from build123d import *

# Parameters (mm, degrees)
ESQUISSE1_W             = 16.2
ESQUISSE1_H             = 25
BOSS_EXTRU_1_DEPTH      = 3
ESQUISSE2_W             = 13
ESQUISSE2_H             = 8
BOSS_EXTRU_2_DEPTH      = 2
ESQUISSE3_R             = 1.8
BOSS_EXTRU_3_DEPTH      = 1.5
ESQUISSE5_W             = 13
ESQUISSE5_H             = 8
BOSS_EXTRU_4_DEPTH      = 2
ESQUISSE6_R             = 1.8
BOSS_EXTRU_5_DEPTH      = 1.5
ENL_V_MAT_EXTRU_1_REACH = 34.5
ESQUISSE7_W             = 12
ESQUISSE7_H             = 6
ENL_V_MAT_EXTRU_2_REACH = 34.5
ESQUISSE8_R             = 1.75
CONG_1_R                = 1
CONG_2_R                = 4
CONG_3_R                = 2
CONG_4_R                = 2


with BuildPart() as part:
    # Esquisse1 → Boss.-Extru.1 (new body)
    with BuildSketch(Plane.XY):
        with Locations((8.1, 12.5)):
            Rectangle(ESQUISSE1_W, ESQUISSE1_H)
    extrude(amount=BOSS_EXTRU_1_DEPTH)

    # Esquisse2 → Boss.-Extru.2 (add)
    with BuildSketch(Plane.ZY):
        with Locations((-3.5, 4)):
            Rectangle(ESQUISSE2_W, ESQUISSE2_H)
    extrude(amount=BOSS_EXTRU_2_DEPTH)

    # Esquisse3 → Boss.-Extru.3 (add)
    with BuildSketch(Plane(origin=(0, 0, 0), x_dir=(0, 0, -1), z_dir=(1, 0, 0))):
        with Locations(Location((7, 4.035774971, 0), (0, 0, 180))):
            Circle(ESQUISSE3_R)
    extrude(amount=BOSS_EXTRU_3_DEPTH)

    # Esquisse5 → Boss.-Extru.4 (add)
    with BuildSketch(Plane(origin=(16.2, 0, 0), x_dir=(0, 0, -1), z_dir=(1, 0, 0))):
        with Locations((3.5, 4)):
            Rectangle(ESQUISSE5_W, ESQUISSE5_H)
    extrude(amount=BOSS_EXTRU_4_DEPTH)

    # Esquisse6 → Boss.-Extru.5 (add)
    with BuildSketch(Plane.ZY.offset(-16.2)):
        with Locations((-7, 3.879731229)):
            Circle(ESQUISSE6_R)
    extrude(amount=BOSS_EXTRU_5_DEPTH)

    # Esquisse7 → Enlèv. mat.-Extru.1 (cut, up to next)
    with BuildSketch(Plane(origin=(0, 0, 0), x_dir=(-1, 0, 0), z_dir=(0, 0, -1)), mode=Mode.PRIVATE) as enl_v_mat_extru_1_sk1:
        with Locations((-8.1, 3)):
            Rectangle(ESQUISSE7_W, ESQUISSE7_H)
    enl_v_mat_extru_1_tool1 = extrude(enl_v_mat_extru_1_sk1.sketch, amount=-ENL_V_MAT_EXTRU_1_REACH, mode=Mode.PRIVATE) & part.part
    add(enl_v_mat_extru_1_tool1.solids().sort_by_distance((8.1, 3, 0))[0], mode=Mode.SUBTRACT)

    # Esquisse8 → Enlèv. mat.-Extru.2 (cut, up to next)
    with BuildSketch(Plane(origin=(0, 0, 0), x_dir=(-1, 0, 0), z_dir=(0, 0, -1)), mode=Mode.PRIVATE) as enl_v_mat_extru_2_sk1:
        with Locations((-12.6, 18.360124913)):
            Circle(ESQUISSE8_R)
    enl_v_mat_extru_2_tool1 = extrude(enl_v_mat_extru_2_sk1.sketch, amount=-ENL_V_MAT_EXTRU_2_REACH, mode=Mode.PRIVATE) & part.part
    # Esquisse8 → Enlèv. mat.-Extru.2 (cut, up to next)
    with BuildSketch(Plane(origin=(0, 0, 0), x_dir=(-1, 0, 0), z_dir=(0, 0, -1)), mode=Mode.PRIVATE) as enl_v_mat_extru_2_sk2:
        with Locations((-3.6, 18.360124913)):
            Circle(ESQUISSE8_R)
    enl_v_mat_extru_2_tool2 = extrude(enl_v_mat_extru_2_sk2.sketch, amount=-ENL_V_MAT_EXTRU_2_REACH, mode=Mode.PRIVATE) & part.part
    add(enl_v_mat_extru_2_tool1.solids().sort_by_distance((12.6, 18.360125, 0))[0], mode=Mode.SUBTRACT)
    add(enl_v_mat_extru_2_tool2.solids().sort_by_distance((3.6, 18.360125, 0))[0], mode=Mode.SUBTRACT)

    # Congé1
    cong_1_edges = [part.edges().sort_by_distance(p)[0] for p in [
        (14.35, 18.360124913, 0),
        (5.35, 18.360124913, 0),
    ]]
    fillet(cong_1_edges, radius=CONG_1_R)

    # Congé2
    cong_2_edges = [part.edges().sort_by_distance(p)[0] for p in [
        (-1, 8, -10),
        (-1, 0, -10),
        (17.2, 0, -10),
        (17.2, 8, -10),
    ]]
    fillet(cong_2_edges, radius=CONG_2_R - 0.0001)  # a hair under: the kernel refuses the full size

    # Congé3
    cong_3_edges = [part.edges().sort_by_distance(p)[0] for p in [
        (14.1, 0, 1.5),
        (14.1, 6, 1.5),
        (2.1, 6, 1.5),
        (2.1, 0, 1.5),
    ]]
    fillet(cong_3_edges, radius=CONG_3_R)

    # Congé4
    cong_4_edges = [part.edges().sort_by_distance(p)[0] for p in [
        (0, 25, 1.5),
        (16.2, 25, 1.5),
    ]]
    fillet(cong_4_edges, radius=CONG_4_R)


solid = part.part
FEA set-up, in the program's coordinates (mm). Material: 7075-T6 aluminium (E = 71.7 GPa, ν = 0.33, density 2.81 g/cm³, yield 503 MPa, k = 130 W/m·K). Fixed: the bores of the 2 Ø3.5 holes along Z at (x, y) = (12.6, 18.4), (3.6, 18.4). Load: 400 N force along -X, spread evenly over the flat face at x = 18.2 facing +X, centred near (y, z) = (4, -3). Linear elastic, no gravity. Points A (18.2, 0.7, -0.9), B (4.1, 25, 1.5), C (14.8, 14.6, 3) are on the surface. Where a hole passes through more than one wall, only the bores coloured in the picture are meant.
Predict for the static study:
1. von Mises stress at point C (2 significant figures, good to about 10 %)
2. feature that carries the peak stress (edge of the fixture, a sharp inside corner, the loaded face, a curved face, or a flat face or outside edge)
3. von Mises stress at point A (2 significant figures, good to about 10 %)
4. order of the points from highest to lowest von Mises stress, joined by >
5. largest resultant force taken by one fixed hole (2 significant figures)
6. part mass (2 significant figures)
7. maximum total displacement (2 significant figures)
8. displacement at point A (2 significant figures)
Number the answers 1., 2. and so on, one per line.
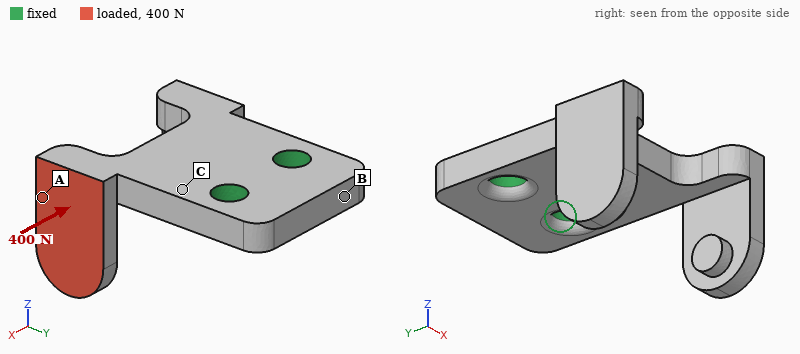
1. 100 MPa
2. a curved face
3. 180 MPa
4. A > C > B
5. 600 N
6. 3.8 g
7. 0.39 mm
8. 0.14 mm
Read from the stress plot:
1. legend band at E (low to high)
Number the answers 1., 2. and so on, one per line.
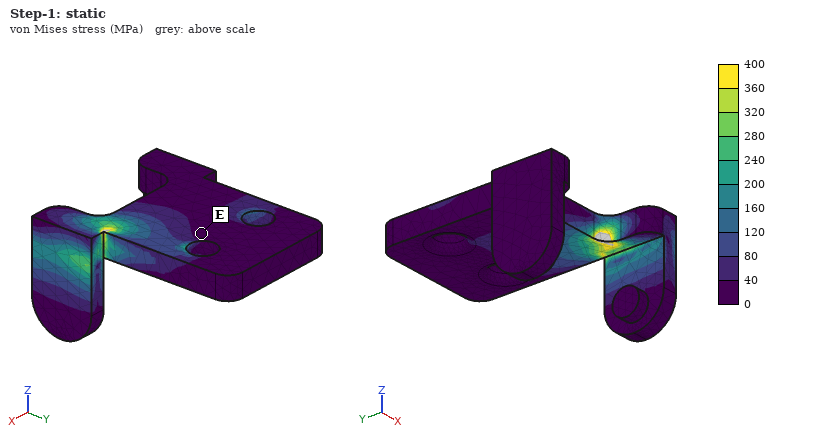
1. 0 to 40 MPa
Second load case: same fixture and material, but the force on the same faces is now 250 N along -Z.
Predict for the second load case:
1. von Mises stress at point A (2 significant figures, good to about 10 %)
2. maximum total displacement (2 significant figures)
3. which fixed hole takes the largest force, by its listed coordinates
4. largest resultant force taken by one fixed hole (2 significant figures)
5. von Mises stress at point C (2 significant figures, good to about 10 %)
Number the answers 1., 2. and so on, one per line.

1. 31 MPa
2. 0.35 mm
3. (12.6, 18.4)
4. 340 N
5. 180 MPa
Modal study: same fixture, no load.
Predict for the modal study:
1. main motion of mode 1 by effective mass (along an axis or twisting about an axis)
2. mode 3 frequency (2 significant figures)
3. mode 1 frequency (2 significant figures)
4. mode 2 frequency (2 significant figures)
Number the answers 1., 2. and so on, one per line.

1. along Z
2. 8200 Hz
3. 5200 Hz
4. 6100 Hz
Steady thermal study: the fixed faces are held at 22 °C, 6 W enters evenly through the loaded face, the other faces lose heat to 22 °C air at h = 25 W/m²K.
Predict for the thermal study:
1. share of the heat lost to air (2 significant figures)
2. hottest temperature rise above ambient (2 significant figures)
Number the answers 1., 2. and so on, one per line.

1. 4.6 %
2. 40 K
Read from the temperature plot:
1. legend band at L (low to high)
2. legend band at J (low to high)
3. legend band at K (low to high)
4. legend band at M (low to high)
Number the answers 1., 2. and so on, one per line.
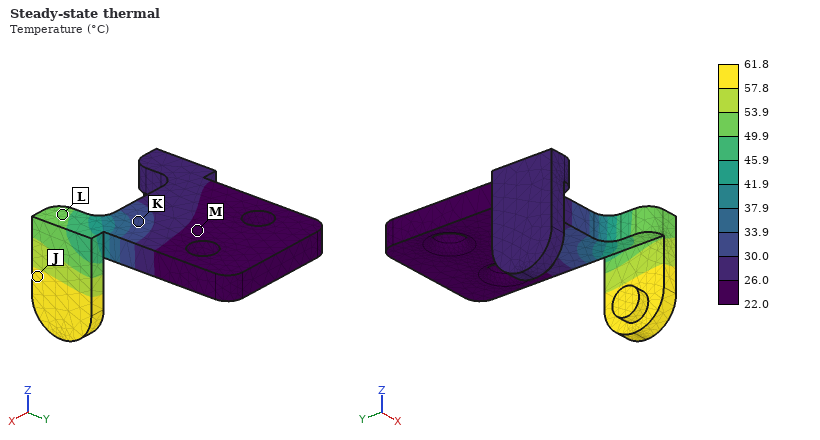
1. 49.9 to 53.9 °C
2. 57.8 to 61.8 °C
3. 30.0 to 33.9 °C
4. 22.0 to 26.0 °C
